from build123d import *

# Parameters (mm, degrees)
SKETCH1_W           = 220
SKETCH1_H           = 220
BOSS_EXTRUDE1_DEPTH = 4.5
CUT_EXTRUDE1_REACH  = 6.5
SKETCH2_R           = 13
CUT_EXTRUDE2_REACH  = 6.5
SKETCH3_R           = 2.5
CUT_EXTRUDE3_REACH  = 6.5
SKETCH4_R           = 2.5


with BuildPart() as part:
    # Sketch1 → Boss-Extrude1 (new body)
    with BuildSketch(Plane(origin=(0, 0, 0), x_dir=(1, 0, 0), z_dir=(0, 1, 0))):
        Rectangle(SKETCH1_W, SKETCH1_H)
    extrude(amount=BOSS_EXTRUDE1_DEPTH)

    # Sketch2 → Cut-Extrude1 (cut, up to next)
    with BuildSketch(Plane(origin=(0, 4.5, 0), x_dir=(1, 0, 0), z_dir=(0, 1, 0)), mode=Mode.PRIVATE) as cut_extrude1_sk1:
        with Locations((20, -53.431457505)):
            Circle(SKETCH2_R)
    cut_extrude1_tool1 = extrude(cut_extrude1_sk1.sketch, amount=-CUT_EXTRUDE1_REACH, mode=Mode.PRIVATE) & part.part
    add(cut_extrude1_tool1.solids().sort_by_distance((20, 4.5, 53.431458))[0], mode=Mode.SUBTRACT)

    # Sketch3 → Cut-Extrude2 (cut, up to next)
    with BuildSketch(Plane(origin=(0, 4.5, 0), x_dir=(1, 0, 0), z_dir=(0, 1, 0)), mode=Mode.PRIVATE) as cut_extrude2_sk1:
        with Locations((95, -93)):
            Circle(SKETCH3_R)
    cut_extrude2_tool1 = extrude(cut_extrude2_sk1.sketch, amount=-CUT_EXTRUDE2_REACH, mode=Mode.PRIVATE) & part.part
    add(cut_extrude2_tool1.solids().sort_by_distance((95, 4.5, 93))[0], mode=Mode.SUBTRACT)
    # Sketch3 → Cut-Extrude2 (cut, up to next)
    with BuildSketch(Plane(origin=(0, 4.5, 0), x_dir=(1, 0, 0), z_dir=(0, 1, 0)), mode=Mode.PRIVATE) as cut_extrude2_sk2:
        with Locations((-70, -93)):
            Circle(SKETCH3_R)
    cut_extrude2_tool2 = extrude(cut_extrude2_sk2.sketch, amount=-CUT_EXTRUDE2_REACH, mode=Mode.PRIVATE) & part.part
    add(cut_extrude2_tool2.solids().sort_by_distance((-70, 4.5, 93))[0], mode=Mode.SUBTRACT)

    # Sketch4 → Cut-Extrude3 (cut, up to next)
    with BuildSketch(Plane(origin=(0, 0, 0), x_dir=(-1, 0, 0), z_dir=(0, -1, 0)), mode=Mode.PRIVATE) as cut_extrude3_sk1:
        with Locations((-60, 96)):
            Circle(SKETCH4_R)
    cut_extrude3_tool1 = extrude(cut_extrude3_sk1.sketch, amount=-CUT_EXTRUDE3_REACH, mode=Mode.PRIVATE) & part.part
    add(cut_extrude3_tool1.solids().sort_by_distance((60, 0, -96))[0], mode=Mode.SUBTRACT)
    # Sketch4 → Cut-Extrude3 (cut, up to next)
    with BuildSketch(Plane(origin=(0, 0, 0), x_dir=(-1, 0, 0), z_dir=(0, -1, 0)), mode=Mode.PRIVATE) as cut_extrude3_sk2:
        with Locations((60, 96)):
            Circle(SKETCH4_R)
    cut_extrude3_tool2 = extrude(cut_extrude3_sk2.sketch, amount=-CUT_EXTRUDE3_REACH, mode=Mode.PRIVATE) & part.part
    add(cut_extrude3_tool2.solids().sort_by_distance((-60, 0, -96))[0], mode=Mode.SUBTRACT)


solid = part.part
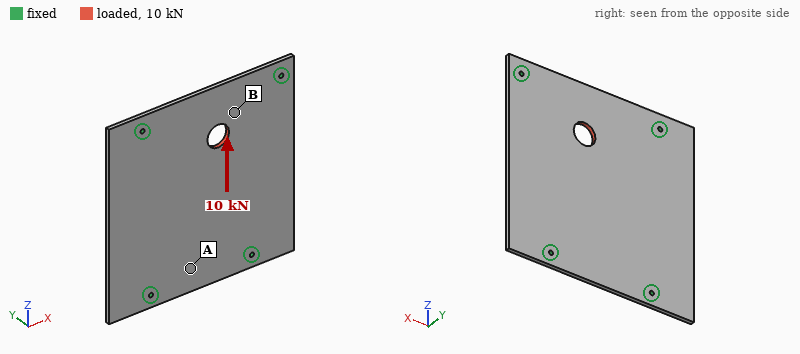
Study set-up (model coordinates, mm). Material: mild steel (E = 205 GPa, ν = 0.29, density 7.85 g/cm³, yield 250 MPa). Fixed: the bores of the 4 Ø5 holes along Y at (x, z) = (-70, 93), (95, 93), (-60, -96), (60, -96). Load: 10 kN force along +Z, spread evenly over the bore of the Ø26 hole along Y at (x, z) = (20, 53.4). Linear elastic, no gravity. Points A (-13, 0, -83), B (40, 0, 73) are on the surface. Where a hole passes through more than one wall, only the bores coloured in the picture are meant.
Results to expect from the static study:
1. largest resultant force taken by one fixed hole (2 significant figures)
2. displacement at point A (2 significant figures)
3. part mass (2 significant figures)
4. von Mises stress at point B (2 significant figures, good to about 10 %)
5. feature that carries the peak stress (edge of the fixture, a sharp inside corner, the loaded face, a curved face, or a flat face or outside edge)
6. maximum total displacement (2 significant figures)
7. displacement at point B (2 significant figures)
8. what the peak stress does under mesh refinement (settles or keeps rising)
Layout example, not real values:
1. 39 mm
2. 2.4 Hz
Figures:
1. 2.9 kN
2. 3.4 µm
3. 1.7 kg
4. 18 MPa
5. edge of the fixture
6. 14 µm
7. 10 µm
8. keeps rising
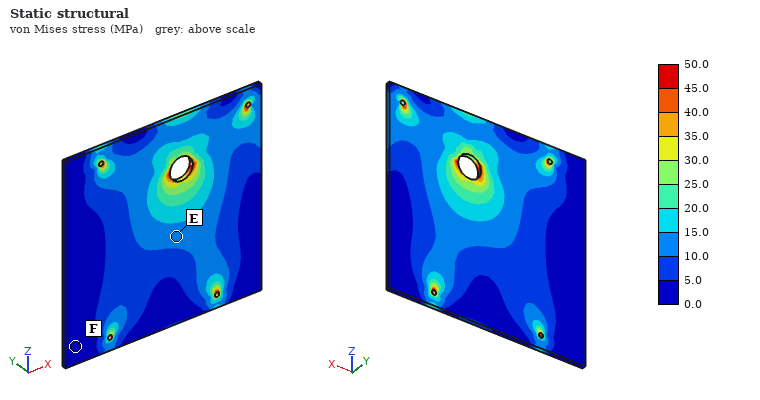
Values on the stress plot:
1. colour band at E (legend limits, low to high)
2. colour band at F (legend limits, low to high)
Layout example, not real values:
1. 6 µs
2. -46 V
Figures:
1. 10.0 to 15.0 MPa
2. 0.0 to 5.0 MPa
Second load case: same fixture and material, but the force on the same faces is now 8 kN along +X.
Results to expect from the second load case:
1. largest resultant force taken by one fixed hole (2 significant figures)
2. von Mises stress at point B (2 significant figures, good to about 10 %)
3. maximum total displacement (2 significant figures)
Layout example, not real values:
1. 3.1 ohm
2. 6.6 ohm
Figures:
1. 3.1 kN
2. 16 MPa
3. 9.0 µm
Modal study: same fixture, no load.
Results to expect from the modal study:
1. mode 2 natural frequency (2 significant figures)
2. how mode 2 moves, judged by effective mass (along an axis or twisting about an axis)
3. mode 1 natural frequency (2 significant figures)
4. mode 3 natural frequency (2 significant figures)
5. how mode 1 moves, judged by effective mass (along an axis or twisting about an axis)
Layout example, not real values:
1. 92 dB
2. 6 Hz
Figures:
1. 620 Hz
2. twisting about Z
3. 490 Hz
4. 760 Hz
5. along Y
